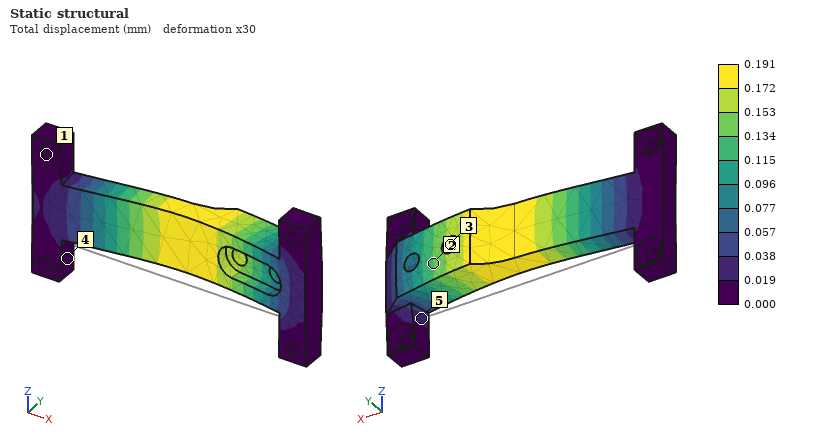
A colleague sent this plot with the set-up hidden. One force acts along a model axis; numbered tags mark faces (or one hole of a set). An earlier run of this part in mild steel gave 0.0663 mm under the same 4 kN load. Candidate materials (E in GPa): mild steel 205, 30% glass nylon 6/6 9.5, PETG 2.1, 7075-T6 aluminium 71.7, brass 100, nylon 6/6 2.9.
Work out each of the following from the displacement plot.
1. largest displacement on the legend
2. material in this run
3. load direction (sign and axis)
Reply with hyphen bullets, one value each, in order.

- 0.191 mm
- 7075-T6 aluminium
- +Y
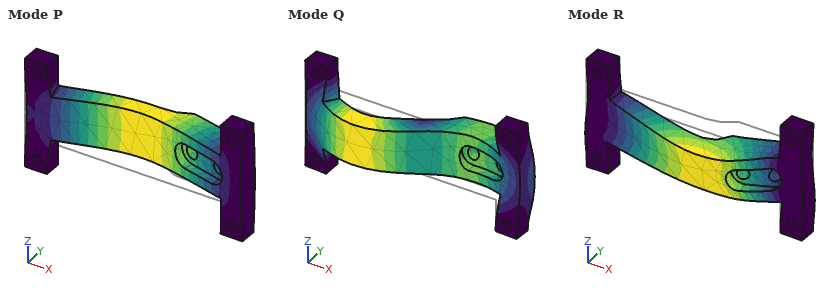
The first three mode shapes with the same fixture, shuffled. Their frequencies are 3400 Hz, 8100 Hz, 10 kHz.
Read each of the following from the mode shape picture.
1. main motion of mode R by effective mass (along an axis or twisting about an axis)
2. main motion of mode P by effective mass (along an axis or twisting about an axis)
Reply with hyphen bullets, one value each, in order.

- along Z
- along Y
